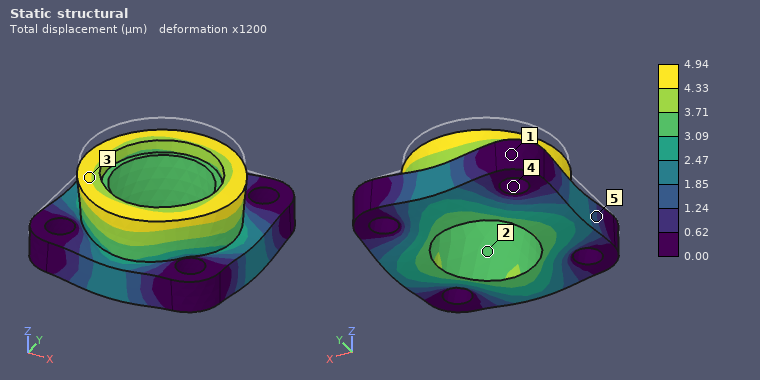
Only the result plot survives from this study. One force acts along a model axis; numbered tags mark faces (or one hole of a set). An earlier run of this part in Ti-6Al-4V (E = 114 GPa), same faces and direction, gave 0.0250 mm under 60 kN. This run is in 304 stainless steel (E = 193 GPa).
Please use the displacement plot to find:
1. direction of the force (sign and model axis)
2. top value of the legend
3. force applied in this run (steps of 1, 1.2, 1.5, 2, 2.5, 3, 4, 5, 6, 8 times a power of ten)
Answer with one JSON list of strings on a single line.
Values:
["-Z", "4.94 µm", "20 kN"]
